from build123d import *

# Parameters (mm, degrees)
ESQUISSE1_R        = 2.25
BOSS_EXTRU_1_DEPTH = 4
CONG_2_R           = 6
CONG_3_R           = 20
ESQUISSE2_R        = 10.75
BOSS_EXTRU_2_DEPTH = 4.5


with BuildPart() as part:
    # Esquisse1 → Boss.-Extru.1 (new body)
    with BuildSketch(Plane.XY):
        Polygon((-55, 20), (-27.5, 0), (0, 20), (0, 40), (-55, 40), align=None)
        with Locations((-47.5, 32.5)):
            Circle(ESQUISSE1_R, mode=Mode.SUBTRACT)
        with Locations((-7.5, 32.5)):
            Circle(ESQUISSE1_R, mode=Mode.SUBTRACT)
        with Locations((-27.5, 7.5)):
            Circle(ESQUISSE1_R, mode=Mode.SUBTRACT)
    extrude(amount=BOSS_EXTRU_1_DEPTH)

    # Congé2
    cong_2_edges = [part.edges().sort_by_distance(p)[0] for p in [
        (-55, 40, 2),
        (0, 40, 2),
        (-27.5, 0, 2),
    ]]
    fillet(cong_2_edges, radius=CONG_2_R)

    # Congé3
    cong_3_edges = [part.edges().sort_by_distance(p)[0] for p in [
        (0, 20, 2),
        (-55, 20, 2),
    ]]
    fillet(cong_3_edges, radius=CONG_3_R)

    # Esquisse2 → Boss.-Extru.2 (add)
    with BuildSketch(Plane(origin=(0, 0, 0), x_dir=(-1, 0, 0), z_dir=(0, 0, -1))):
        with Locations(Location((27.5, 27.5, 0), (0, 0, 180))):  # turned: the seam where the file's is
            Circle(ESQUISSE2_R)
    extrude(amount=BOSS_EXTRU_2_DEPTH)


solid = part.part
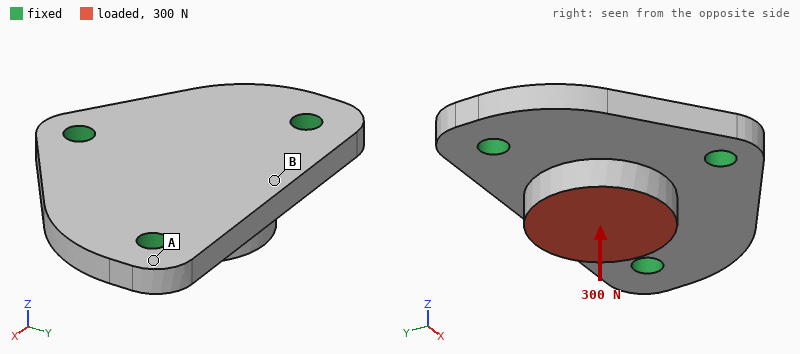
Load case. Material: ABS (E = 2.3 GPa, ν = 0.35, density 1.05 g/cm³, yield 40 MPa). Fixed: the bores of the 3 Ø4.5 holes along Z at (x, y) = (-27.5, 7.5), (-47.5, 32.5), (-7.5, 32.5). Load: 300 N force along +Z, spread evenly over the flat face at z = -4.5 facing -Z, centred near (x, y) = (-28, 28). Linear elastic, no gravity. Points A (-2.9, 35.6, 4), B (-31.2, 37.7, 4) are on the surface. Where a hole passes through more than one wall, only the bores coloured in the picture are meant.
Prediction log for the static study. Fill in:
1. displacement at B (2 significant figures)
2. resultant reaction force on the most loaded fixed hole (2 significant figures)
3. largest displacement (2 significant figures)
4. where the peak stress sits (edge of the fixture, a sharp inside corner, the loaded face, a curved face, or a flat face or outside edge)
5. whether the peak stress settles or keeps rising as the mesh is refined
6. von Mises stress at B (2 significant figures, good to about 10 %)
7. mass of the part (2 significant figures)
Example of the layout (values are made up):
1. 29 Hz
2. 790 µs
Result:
1. 0.14 mm
2. 120 N
3. 0.15 mm
4. edge of the fixture
5. keeps rising
6. 5.2 MPa
7. 8.2 g
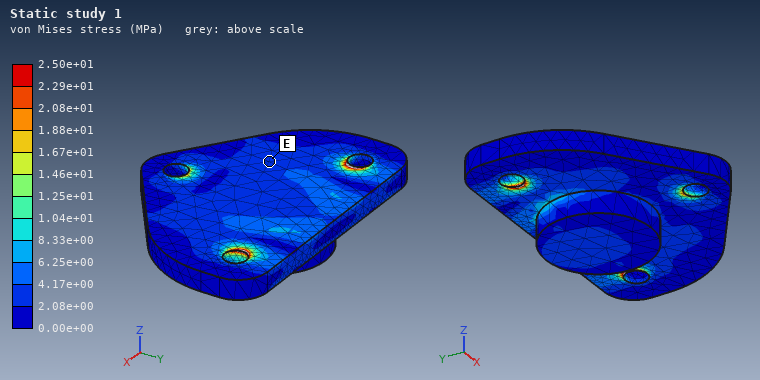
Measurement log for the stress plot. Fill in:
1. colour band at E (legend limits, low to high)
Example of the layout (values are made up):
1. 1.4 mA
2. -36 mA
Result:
1. 2.08e+00 to 4.17e+00 MPa
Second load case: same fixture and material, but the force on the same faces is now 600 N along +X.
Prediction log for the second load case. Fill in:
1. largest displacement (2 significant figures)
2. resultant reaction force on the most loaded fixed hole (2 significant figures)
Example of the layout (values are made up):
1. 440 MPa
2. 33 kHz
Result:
1. 0.10 mm
2. 270 N
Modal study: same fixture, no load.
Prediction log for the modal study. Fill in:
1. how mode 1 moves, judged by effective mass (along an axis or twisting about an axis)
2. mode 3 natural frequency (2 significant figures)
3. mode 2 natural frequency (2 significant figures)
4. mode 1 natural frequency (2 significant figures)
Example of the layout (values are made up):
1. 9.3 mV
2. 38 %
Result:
1. along Z
2. 5400 Hz
3. 5300 Hz
4. 4100 Hz
